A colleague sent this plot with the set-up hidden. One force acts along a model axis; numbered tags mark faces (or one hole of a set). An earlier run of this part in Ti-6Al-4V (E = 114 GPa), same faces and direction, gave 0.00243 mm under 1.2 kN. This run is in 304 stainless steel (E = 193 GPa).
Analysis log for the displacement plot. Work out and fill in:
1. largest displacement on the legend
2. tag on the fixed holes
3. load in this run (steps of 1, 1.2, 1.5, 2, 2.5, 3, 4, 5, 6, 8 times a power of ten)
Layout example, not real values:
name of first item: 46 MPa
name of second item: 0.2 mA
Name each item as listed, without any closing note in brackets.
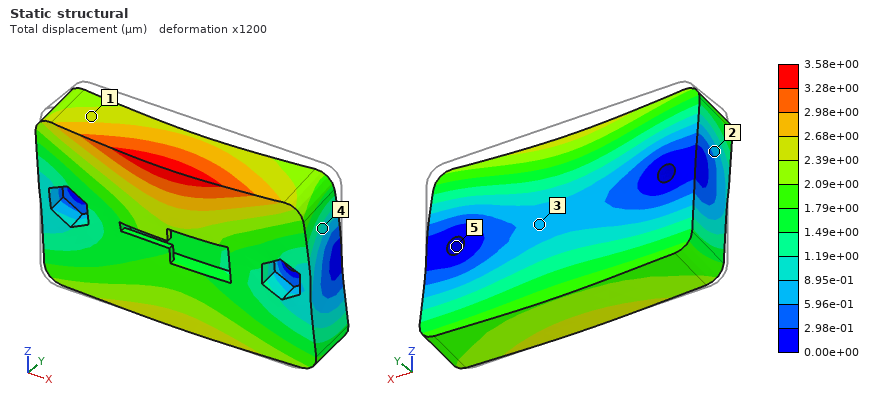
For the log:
largest displacement on the legend: 3.58e+00 µm
tag on the fixed holes: 5
load in this run: 3 kN
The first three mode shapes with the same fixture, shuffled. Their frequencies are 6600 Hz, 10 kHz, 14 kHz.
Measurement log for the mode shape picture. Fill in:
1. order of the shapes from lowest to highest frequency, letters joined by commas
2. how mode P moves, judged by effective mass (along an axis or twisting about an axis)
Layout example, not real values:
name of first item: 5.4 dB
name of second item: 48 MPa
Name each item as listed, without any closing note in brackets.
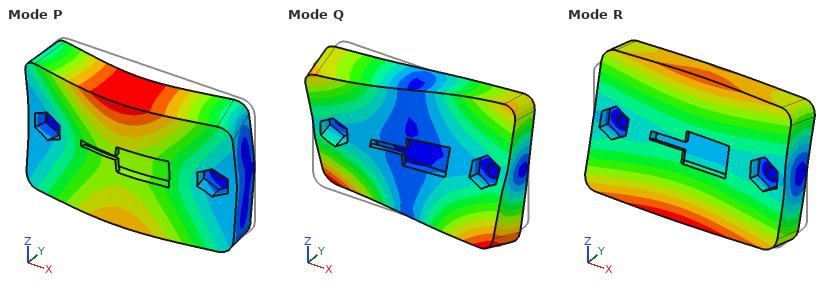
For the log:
order of the shapes from lowest to highest frequency, letters joined by commas: R, P, Q
how mode P moves, judged by effective mass: along Y
